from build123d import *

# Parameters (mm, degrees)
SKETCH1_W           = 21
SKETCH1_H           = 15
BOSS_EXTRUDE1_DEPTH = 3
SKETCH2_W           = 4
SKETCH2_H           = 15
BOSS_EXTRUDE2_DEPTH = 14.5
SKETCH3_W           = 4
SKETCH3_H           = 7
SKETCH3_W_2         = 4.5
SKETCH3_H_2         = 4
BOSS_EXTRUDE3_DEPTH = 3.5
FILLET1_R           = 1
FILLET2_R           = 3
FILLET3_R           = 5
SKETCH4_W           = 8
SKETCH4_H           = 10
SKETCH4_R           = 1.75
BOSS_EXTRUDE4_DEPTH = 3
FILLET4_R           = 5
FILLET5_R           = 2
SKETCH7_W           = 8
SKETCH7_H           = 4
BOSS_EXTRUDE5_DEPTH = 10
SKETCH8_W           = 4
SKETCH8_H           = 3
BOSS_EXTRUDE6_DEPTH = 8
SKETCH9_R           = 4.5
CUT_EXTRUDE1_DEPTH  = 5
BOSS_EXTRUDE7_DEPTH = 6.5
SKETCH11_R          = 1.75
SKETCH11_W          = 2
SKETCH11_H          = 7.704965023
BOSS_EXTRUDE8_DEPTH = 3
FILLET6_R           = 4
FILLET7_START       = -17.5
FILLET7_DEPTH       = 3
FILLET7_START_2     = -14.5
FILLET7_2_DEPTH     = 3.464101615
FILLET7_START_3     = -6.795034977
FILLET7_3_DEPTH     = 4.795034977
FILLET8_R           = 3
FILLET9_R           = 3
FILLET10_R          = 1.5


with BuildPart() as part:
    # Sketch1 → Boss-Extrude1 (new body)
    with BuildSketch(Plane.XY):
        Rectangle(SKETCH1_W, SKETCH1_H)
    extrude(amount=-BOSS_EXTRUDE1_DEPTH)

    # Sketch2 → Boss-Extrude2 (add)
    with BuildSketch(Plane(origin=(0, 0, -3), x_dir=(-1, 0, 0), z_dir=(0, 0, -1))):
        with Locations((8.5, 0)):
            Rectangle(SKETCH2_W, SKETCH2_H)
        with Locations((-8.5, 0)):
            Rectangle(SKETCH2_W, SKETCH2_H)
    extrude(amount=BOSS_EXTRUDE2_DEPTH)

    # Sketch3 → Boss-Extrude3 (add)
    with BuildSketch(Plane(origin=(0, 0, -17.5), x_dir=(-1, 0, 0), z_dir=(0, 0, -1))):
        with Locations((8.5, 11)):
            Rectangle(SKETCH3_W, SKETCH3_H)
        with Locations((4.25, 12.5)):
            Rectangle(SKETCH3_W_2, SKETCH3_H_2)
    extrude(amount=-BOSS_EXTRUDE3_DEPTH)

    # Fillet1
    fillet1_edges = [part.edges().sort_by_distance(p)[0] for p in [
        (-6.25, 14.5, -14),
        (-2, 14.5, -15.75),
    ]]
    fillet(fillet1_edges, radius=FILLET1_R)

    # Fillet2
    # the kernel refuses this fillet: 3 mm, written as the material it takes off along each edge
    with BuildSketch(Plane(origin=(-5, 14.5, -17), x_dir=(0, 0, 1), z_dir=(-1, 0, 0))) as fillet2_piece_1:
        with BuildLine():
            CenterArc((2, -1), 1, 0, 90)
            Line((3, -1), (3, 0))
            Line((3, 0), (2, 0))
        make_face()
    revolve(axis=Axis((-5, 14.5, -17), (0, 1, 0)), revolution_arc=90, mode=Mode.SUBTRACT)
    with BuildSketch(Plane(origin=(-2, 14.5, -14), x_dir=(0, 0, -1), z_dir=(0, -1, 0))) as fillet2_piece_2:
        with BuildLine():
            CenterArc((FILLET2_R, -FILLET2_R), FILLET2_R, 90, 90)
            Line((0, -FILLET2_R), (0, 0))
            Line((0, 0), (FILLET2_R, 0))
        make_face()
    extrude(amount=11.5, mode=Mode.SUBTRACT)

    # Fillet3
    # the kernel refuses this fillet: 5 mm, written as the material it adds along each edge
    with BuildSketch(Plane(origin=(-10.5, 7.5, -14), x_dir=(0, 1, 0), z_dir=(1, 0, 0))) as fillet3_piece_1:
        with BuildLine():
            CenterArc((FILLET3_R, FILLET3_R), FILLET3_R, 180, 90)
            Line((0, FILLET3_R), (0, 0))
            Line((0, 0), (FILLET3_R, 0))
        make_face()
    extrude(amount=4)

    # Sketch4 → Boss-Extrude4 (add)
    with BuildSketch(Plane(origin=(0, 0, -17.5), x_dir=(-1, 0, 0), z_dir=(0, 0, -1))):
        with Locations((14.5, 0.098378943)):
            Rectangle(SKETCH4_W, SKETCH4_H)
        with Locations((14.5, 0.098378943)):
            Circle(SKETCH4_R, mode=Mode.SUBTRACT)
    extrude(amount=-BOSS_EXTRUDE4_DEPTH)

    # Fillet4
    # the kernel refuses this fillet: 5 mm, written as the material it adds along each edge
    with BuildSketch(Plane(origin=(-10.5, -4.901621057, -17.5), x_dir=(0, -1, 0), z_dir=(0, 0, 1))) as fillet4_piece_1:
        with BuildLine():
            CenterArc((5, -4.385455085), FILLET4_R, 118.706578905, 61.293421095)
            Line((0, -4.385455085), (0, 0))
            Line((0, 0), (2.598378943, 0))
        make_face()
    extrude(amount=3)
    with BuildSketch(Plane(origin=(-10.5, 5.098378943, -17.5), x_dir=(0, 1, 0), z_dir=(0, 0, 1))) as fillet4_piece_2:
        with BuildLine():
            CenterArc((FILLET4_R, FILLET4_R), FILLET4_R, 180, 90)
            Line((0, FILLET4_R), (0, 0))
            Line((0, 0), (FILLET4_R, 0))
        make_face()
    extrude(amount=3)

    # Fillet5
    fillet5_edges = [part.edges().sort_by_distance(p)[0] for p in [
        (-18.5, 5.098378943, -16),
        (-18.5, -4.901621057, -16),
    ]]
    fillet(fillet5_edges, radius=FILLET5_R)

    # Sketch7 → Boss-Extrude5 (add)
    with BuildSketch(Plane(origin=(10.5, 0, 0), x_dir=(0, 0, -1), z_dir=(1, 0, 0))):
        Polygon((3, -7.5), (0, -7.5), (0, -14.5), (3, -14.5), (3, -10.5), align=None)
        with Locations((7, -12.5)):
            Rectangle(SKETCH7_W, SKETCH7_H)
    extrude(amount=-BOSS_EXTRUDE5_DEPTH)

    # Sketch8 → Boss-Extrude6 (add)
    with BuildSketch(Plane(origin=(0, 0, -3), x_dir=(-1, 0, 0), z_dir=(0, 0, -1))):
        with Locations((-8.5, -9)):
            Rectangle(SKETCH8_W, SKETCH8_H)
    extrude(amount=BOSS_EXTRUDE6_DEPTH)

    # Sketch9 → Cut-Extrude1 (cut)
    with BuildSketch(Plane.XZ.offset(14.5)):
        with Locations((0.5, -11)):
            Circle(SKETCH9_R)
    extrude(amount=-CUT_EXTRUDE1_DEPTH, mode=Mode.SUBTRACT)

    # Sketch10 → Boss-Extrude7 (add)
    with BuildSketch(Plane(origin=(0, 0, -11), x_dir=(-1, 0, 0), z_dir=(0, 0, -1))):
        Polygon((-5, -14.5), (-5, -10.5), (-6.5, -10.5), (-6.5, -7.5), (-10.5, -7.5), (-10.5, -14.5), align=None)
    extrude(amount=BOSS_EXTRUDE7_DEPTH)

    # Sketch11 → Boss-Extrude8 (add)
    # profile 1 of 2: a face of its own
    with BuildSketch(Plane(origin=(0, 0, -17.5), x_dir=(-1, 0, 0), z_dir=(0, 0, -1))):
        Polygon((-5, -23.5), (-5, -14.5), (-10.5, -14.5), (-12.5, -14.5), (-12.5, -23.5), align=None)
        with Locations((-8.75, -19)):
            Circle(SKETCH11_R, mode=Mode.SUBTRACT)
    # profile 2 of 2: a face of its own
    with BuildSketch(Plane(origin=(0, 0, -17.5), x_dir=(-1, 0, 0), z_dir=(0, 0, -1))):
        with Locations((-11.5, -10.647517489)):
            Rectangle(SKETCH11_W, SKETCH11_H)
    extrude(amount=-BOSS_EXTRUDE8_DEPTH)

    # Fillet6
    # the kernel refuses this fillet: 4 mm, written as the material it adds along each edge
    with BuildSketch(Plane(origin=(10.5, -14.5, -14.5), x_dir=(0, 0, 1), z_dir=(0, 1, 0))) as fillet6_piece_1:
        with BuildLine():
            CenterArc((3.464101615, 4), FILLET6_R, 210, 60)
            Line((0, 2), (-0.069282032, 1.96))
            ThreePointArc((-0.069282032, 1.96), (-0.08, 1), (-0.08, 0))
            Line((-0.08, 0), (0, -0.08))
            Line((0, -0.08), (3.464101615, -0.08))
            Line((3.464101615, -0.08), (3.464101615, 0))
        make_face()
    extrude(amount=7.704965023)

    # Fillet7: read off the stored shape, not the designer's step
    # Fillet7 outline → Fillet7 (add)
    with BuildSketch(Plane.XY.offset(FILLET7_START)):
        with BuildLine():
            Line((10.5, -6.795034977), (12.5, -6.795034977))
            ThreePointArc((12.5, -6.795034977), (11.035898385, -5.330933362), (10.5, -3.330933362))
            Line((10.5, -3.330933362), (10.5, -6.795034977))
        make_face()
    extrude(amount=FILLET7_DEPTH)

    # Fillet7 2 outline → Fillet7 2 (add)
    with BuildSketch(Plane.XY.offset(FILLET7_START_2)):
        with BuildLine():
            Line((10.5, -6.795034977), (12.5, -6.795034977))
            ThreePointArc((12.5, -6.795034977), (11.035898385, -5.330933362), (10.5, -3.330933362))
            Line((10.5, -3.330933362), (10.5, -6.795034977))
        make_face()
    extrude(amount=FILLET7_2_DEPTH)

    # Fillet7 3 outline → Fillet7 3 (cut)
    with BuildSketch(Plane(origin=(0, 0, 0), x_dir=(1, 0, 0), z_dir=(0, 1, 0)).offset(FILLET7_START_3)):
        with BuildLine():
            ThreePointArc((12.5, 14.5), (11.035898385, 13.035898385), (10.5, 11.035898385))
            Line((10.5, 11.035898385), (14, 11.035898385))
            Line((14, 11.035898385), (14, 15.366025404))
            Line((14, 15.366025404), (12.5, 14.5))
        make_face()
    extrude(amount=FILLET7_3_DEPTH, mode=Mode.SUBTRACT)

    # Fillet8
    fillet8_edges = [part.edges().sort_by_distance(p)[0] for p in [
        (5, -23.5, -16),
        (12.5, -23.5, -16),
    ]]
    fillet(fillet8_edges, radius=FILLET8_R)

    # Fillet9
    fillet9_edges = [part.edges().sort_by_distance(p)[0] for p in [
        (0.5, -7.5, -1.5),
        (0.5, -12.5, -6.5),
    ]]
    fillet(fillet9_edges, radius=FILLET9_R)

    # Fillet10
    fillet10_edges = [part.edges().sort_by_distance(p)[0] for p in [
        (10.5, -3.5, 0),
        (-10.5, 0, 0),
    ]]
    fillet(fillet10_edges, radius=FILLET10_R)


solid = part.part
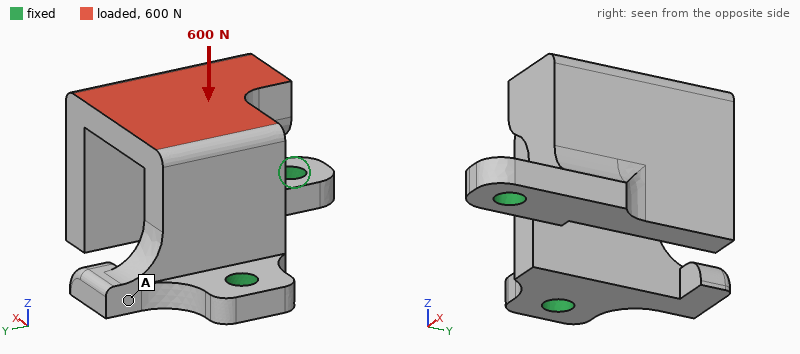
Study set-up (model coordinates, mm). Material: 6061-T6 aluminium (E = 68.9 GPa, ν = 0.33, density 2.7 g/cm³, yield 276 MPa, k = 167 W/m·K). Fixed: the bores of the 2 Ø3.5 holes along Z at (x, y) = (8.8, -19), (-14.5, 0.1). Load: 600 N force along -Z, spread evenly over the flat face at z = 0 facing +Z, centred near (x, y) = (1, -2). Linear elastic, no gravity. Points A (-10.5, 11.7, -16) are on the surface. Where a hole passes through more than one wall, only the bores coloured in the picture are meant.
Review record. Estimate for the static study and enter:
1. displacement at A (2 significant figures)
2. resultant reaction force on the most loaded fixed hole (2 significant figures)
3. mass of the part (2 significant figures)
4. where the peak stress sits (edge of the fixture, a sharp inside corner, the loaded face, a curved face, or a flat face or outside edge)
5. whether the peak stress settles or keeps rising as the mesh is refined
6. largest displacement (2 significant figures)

0.039 mm
350 N
11 g
edge of the fixture
keeps rising
0.13 mm
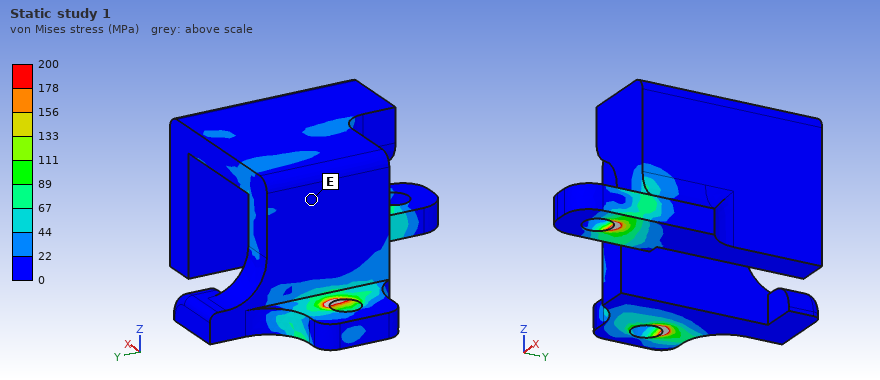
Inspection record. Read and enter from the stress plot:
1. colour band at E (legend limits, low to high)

0 to 22 MPa
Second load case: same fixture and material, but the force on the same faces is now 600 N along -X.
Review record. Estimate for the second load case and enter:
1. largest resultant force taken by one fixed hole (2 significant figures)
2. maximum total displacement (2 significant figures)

460 N
0.17 mm
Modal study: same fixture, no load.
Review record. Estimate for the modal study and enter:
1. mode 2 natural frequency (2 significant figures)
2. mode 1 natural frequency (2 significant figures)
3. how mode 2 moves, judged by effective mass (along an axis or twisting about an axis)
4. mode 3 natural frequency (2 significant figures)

6800 Hz
3400 Hz
along X
10 kHz
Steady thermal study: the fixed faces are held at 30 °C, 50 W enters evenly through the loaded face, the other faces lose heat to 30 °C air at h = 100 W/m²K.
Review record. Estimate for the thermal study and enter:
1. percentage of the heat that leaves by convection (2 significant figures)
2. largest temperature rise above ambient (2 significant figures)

18 %
62 K
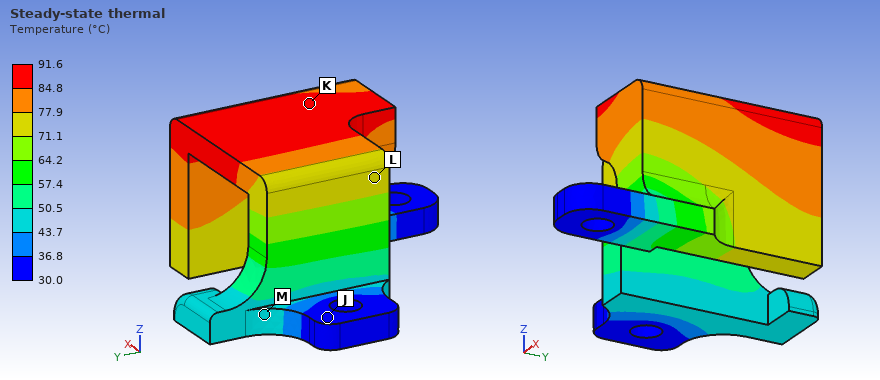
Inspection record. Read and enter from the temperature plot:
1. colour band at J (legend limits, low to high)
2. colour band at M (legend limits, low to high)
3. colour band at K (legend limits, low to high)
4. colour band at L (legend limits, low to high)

30.0 to 36.8 °C
43.7 to 50.5 °C
84.8 to 91.6 °C
71.1 to 77.9 °C
